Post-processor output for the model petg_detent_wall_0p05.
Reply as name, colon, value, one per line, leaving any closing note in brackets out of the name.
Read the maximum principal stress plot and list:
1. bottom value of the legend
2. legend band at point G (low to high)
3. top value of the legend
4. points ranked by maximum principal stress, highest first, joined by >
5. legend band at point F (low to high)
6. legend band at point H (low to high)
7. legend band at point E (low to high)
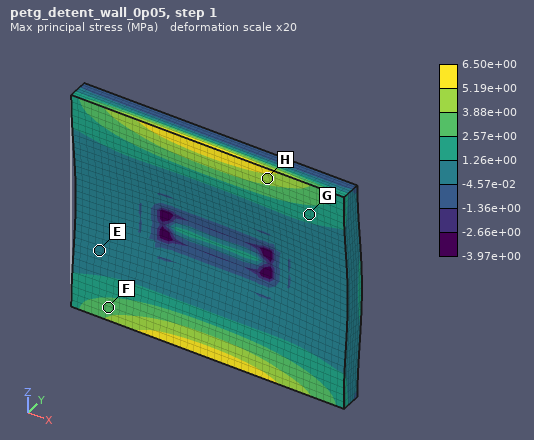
bottom value of the legend: -3.97e+00 MPa
legend band at point G: 1.26e+00 to 2.57e+00 MPa
top value of the legend: 6.50e+00 MPa
points ranked by maximum principal stress, highest first, joined by >: H > F > G > E
legend band at point F: 2.57e+00 to 3.88e+00 MPa
legend band at point H: 3.88e+00 to 5.19e+00 MPa
legend band at point E: -4.57e-02 to 1.26e+00 MPa
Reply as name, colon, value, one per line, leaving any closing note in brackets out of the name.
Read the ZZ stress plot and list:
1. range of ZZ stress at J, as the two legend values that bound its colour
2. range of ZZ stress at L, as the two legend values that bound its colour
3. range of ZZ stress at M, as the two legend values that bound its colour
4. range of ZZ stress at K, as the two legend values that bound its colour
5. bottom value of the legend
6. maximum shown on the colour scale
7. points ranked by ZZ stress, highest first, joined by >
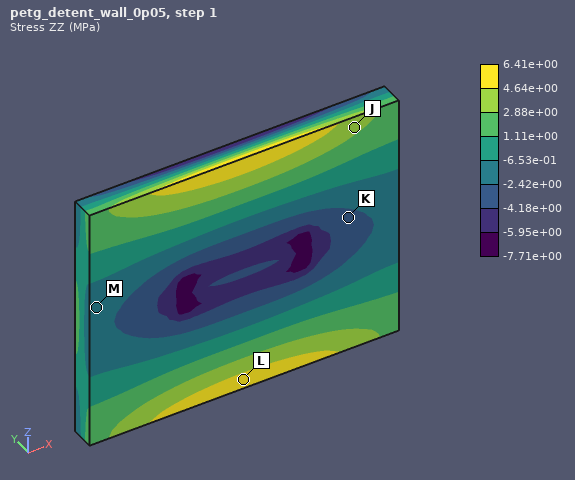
range of ZZ stress at J, as the two legend values that bound its colour: 2.88e+00 to 4.64e+00 MPa
range of ZZ stress at L, as the two legend values that bound its colour: 4.64e+00 to 6.41e+00 MPa
range of ZZ stress at M, as the two legend values that bound its colour: -2.42e+00 to -6.53e-01 MPa
range of ZZ stress at K, as the two legend values that bound its colour: -4.18e+00 to -2.42e+00 MPa
bottom value of the legend: -7.71e+00 MPa
maximum shown on the colour scale: 6.41e+00 MPa
points ranked by ZZ stress, highest first, joined by >: L > J > M > K
